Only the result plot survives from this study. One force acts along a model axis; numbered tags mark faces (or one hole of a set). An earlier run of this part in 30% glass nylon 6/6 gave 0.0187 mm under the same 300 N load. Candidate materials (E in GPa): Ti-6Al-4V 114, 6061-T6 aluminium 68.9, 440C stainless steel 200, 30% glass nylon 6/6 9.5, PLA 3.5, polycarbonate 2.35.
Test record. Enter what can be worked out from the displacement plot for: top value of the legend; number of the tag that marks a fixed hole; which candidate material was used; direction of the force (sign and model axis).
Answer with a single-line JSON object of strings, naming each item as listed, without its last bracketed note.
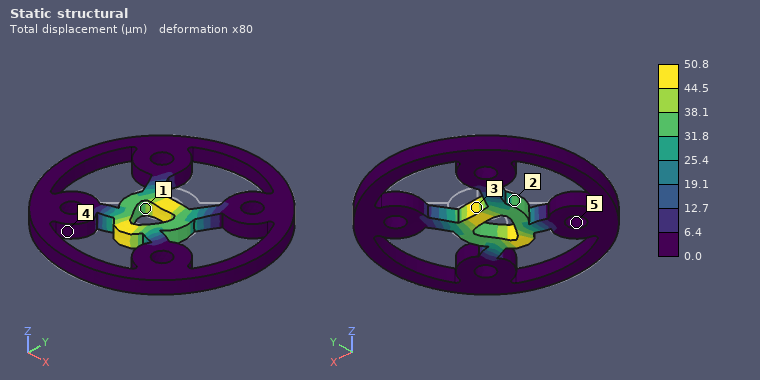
{"top value of the legend": "50.8 µm", "number of the tag that marks a fixed hole": "5", "which candidate material was used": "PLA", "direction of the force": "-Y"}
